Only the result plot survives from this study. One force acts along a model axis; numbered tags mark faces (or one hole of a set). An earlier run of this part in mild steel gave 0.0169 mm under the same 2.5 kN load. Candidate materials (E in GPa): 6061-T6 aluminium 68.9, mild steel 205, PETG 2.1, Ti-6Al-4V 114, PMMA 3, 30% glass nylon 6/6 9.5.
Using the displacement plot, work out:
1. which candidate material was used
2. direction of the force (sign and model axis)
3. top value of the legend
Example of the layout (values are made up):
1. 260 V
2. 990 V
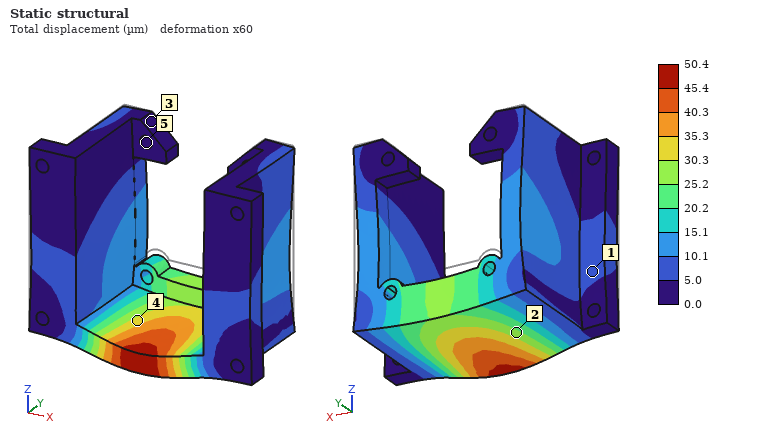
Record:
1. 6061-T6 aluminium
2. -Z
3. 50.4 µm
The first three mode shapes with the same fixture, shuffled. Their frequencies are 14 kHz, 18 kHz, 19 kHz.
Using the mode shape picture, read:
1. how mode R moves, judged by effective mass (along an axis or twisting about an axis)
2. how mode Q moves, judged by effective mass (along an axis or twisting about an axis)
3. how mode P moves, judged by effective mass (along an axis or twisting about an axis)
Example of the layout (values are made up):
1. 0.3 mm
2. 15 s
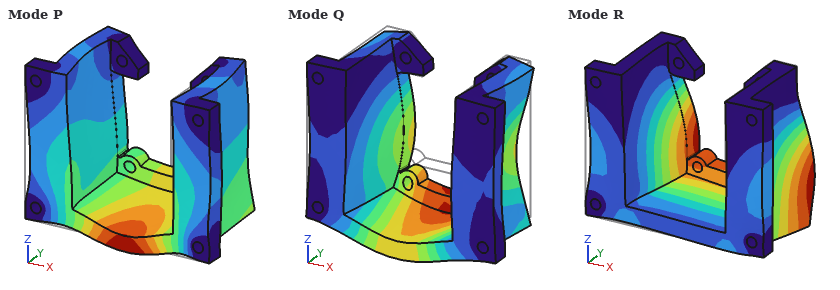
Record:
1. along X
2. along Z
3. along Y
